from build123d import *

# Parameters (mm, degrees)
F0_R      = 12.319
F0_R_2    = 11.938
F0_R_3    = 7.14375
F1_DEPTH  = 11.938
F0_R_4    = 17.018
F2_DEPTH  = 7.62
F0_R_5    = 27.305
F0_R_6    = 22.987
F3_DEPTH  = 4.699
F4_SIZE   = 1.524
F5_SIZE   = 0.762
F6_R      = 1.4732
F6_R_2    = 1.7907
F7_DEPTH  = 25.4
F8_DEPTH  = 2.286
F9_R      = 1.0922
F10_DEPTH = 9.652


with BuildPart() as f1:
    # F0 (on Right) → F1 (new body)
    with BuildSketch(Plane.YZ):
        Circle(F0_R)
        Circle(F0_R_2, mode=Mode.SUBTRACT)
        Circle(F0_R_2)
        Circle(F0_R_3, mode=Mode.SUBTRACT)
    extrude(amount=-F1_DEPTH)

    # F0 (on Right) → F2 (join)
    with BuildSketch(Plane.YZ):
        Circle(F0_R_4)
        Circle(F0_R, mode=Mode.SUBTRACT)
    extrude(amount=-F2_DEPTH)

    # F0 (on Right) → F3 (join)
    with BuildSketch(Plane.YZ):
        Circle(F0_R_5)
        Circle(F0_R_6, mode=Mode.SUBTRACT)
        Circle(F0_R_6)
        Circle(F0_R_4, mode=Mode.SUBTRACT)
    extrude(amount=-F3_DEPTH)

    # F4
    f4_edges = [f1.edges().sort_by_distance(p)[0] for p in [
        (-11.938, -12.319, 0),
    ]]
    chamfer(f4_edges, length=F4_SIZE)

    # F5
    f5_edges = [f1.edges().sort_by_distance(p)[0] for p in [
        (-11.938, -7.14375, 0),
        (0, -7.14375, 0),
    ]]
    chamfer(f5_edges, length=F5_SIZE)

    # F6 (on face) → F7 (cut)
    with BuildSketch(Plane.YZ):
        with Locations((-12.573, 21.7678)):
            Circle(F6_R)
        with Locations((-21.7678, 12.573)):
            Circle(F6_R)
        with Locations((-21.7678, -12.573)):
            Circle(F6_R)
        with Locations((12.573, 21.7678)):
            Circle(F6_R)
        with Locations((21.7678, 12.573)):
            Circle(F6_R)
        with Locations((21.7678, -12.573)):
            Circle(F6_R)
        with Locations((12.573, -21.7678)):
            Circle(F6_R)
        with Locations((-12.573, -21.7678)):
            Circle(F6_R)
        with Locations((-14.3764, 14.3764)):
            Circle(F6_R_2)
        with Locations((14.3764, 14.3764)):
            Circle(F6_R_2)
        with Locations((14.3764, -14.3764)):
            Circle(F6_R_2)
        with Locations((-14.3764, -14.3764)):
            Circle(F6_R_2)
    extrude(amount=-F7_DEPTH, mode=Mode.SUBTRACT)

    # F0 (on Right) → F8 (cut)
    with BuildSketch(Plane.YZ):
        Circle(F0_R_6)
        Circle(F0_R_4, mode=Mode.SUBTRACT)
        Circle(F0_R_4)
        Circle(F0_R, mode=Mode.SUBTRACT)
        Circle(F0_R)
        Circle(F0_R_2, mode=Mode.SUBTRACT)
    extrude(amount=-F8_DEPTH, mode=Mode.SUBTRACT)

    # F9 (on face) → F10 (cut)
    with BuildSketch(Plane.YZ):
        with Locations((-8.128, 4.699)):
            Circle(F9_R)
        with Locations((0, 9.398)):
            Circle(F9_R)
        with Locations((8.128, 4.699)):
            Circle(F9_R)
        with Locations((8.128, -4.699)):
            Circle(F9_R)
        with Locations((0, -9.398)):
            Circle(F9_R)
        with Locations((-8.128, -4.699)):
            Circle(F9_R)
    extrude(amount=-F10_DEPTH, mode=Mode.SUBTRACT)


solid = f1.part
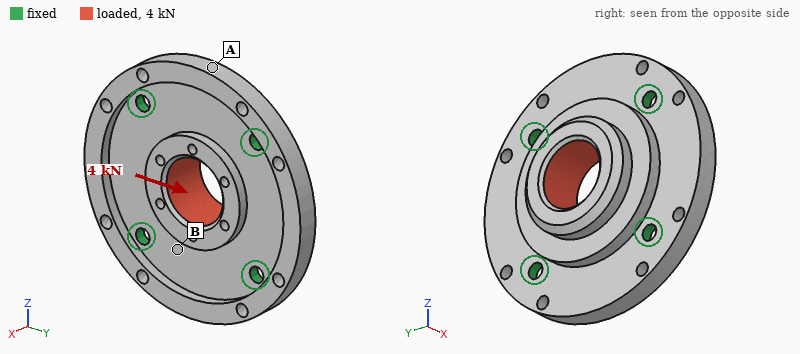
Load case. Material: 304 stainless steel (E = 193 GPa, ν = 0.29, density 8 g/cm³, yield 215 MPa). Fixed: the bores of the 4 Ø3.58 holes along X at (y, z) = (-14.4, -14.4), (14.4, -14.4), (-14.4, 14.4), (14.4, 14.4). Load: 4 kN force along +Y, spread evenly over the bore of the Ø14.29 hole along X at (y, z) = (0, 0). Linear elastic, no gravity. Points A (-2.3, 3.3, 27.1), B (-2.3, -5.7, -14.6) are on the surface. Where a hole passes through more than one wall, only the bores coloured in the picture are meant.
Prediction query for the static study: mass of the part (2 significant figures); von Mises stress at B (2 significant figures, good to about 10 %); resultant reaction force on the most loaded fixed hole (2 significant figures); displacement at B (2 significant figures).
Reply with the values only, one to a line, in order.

83 g
16 MPa
1.0 kN
0.90 µm
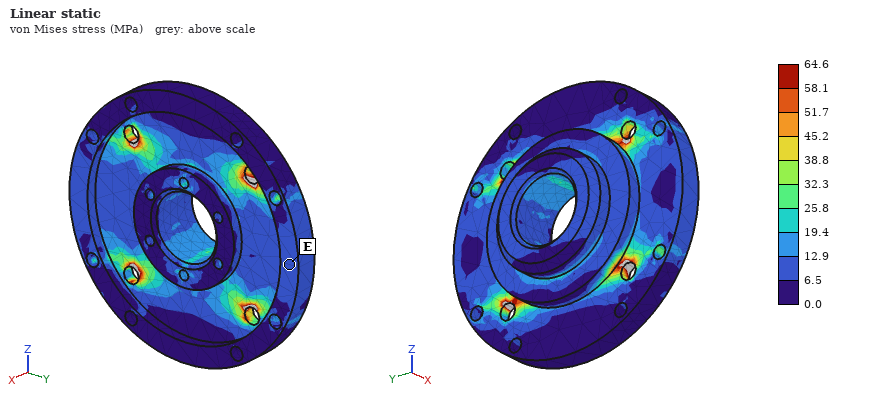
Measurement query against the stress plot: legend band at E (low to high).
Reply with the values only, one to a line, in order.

6.5 to 12.9 MPa
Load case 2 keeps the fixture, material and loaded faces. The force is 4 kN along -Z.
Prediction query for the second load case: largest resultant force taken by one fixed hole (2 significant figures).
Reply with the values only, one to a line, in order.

1.0 kN
